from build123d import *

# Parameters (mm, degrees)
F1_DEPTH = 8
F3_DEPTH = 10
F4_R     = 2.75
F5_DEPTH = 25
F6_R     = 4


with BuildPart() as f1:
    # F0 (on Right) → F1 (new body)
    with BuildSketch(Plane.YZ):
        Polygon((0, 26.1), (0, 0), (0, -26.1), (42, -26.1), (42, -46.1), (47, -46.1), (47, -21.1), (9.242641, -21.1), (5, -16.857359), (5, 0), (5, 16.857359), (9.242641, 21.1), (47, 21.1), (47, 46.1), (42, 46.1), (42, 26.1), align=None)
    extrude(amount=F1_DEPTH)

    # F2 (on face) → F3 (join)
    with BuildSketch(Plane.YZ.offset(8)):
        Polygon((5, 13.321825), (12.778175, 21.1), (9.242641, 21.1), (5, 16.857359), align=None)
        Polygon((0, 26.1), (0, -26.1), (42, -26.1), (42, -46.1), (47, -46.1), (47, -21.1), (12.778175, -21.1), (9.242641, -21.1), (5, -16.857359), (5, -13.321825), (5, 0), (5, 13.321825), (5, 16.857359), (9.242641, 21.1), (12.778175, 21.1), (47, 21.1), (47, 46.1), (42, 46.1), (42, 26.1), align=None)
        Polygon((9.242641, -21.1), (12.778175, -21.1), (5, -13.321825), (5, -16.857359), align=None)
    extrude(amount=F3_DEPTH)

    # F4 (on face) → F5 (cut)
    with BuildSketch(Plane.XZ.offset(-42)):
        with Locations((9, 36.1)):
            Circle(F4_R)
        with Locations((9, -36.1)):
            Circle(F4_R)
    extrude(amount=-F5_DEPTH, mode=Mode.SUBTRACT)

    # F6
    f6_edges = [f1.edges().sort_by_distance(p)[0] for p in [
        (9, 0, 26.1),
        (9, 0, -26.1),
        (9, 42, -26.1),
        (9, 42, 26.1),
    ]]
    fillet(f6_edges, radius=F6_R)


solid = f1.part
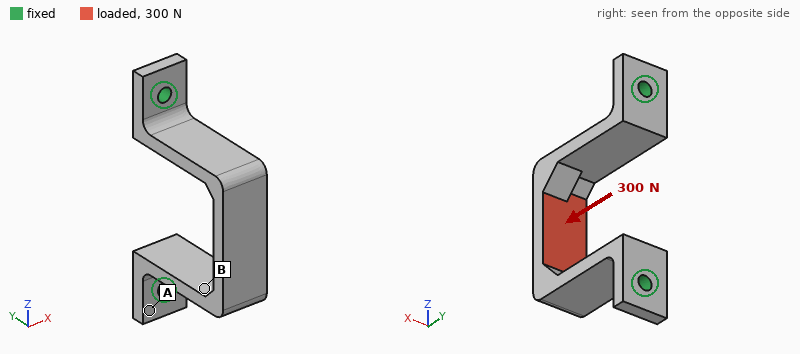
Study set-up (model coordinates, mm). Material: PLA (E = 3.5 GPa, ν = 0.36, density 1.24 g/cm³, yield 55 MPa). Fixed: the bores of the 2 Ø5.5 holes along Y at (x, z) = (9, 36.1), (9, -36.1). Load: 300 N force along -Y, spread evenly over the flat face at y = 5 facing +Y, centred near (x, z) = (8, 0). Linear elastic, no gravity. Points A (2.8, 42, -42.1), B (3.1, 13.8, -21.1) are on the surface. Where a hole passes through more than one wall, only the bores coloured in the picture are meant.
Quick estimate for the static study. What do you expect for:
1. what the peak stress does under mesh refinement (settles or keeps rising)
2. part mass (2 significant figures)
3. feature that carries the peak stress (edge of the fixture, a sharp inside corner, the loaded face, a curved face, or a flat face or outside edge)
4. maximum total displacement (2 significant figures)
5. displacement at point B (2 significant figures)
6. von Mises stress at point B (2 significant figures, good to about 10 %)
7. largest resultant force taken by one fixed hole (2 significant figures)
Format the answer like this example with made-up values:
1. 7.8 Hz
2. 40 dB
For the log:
1. keeps rising
2. 20 g
3. edge of the fixture
4. 0.32 mm
5. 0.11 mm
6. 11 MPa
7. 160 N
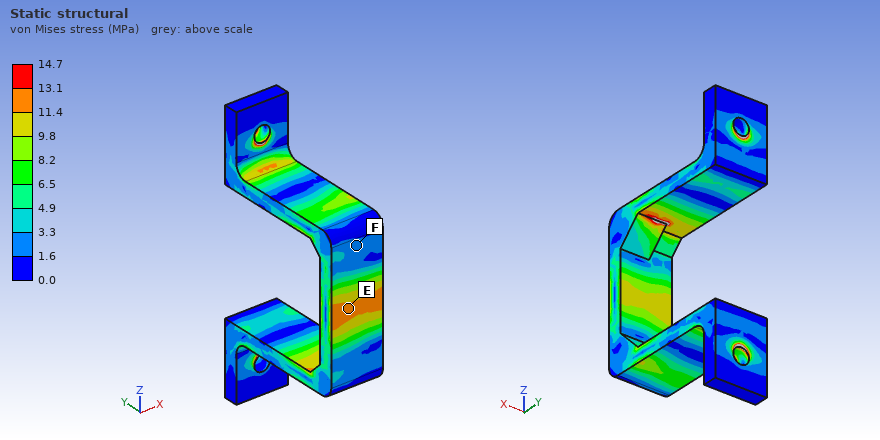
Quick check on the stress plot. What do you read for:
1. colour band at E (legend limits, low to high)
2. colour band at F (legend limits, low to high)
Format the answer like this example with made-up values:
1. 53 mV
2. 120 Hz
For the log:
1. 11.4 to 13.1 MPa
2. 1.6 to 3.3 MPa
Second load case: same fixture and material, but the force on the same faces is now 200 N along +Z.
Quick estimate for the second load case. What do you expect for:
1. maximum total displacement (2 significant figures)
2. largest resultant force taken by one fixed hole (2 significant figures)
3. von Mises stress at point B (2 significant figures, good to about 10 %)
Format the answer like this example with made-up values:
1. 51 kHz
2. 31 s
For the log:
1. 1.0 mm
2. 140 N
3. 14 MPa
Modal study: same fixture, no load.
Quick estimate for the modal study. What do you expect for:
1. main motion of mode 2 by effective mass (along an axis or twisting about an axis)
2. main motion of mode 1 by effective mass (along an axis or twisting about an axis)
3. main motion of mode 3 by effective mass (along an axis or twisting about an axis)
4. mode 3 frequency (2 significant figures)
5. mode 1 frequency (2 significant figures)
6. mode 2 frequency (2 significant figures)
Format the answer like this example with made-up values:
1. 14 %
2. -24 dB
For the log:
1. along Z
2. along X
3. twisting about Y
4. 1000 Hz
5. 560 Hz
6. 740 Hz
